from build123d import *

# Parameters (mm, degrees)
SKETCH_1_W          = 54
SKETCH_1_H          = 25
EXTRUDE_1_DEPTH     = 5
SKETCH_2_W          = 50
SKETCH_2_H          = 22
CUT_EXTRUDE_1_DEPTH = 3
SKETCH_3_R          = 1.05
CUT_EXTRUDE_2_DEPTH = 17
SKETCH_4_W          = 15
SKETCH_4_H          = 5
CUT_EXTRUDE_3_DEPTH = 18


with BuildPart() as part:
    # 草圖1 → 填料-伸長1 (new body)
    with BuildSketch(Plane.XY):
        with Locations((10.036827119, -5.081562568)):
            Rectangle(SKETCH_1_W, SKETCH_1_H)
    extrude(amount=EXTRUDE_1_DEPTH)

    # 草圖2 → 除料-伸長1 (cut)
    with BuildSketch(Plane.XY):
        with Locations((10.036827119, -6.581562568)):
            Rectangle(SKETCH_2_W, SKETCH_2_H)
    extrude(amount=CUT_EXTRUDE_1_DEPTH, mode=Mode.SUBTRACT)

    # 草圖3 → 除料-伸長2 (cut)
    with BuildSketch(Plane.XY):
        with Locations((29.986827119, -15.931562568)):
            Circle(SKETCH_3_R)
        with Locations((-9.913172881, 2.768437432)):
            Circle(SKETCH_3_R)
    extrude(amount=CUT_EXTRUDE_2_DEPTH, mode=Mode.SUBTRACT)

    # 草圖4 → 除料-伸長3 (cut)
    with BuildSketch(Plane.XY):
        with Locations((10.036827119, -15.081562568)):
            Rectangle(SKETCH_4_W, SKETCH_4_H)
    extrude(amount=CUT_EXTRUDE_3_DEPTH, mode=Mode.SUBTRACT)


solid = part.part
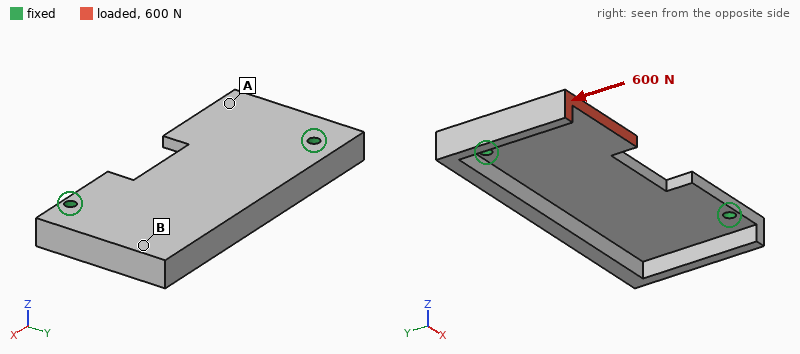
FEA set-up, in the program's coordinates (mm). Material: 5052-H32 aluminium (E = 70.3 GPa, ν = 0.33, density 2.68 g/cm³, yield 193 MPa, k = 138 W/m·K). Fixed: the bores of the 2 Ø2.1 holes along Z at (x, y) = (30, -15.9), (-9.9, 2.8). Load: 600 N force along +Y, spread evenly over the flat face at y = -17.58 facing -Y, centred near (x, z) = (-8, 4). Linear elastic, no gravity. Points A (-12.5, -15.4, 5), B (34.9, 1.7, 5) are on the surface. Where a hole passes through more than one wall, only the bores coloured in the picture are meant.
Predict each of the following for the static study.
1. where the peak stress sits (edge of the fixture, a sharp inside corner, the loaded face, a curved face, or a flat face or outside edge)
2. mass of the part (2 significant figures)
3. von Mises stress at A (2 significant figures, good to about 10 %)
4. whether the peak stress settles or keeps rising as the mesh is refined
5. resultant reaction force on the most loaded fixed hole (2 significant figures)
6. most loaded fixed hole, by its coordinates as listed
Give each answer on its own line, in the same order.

edge of the fixture
8.8 g
13 MPa
keeps rising
560 N
(-9.9, 2.8)
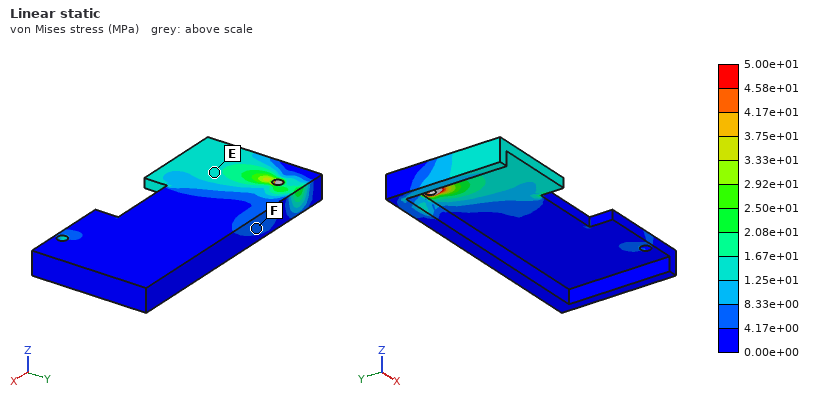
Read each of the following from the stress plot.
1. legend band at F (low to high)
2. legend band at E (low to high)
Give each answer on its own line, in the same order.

4.17e+00 to 8.33e+00 MPa
1.25e+01 to 1.67e+01 MPa
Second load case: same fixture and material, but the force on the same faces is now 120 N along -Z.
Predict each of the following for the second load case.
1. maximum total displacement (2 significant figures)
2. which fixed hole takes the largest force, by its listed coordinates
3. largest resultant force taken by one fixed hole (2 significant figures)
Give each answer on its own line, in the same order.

0.21 mm
(-9.9, 2.8)
110 N
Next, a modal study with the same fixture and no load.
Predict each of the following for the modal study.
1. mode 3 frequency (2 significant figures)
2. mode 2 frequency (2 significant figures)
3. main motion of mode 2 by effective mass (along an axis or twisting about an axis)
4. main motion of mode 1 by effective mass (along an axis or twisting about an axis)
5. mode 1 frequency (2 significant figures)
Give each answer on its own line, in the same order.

6700 Hz
4400 Hz
along Z
along Z
3000 Hz
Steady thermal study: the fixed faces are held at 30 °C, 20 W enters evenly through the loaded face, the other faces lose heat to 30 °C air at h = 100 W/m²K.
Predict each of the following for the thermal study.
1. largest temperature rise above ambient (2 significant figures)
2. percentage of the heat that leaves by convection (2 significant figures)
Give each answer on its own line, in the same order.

61 K
26 %
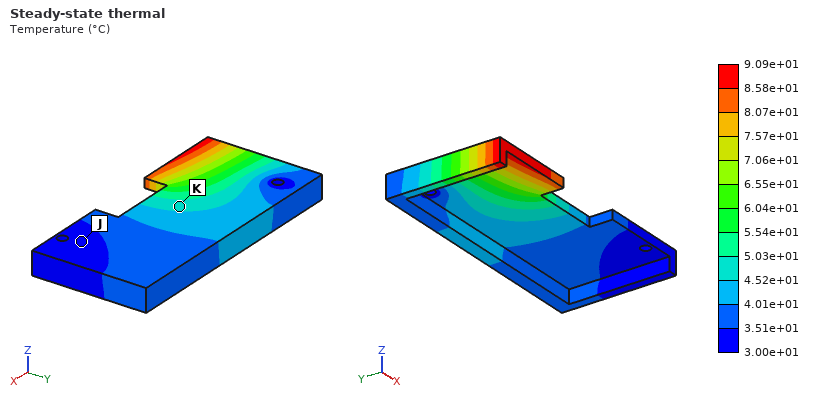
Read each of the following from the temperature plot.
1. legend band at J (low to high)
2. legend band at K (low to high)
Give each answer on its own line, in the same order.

3.00e+01 to 3.51e+01 °C
4.52e+01 to 5.03e+01 °C
